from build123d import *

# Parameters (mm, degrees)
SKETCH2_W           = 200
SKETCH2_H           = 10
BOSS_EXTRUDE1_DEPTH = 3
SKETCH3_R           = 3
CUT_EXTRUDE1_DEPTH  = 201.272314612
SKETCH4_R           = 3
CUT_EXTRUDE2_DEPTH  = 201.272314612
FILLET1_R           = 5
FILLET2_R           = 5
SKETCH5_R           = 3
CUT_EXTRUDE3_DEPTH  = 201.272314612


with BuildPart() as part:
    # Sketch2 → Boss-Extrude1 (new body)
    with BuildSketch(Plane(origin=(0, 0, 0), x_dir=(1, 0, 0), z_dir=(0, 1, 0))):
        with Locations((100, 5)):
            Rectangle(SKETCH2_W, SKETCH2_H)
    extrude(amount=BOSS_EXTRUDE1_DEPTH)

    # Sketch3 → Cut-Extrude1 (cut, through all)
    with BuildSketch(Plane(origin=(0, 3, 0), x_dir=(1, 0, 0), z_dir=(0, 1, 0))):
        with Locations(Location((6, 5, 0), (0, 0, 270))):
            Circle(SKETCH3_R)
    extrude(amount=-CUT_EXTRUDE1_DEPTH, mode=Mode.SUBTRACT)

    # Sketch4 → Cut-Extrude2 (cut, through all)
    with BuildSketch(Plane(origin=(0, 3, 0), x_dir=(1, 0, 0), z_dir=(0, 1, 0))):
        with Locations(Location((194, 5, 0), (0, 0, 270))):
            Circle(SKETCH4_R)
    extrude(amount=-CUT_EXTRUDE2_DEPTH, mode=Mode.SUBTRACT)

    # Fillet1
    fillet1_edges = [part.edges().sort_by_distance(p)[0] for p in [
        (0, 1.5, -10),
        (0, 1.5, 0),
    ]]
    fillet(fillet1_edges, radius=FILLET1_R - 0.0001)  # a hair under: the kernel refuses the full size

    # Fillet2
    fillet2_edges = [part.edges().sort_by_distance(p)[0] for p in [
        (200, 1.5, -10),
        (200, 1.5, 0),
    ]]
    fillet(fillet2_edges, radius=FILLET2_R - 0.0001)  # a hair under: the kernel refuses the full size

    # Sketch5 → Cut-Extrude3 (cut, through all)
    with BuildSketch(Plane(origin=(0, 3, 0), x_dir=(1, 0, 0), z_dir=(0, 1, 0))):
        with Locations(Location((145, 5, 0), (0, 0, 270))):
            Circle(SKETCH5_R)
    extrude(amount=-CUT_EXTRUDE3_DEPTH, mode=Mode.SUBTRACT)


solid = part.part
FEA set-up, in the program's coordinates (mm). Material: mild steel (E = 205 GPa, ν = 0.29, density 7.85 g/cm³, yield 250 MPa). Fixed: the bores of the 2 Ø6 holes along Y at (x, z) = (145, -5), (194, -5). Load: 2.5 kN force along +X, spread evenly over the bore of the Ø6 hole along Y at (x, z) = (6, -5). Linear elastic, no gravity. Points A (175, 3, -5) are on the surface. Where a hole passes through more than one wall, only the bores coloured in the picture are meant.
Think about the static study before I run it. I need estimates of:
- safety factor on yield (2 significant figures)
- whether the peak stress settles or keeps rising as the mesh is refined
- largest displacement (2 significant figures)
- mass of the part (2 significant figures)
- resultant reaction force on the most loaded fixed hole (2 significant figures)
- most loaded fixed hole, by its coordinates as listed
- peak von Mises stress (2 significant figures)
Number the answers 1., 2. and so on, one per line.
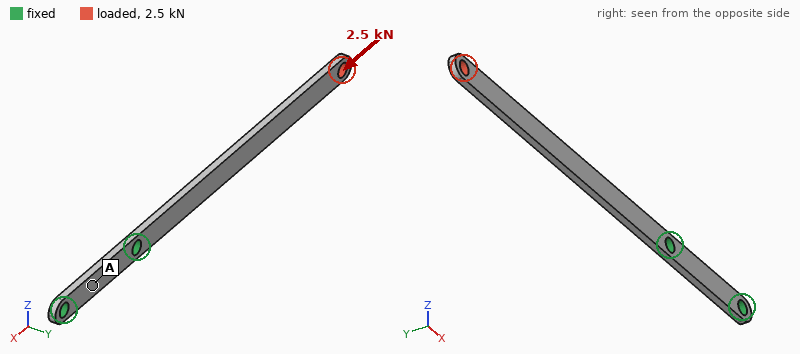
1. 0.93
2. settles
3. 62 µm
4. 45 g
5. 2.5 kN
6. (145, -5)
7. 270 MPa
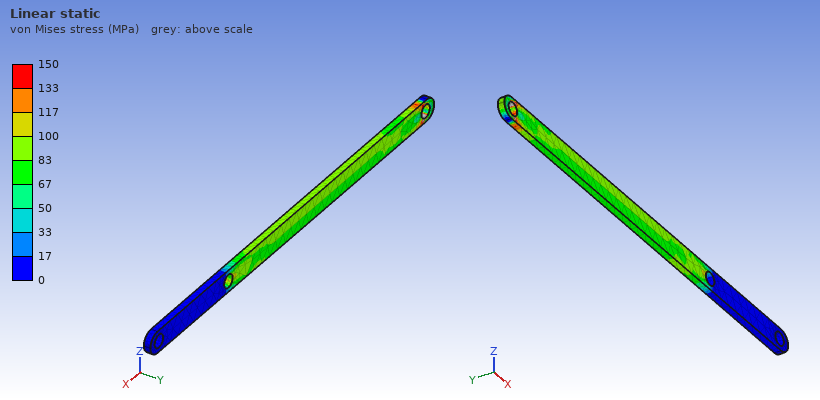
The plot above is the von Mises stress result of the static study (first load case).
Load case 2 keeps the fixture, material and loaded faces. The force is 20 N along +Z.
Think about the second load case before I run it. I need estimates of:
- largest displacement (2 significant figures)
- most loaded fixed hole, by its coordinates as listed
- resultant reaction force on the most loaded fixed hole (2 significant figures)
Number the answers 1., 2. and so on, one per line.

1. 0.37 mm
2. (145, -5)
3. 23 N
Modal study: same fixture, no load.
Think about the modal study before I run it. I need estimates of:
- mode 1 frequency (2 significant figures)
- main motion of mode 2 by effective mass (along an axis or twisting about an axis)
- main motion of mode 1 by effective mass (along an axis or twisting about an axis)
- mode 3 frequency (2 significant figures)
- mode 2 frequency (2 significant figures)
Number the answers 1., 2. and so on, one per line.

1. 130 Hz
2. along Z
3. along Y
4. 800 Hz
5. 410 Hz
